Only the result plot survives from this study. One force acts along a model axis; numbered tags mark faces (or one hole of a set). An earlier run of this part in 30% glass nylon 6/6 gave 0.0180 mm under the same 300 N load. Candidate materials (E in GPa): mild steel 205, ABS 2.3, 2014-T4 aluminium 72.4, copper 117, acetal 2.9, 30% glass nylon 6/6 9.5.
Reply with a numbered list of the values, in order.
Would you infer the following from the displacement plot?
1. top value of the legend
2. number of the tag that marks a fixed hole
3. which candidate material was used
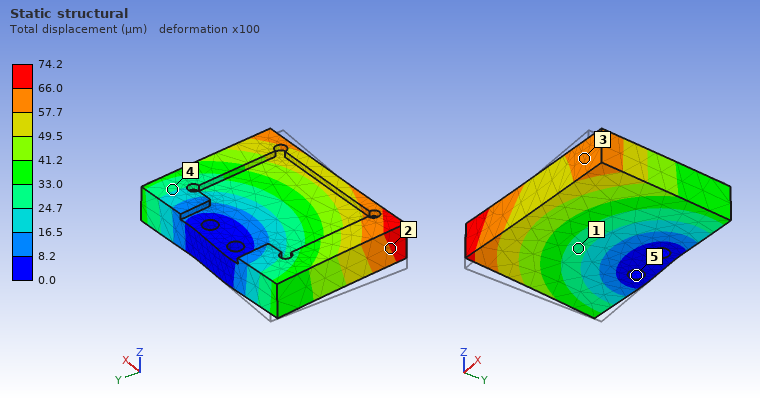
1. 74.2 µm
2. 5
3. ABS
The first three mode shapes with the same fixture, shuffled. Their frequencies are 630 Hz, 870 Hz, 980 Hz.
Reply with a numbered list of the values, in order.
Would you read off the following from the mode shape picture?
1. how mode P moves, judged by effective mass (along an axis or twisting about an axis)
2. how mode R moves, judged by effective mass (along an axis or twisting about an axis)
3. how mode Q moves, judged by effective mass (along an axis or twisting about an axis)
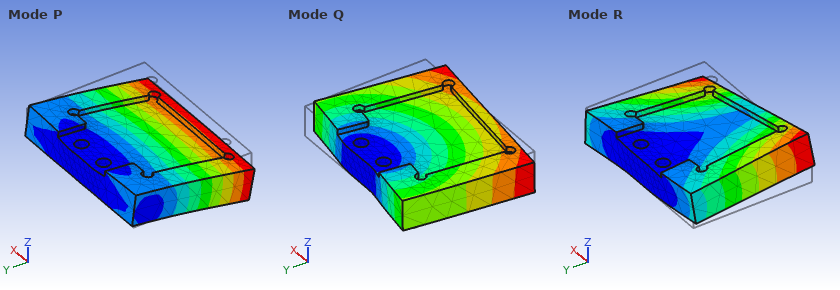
1. along Z
2. twisting about Y
3. along X
